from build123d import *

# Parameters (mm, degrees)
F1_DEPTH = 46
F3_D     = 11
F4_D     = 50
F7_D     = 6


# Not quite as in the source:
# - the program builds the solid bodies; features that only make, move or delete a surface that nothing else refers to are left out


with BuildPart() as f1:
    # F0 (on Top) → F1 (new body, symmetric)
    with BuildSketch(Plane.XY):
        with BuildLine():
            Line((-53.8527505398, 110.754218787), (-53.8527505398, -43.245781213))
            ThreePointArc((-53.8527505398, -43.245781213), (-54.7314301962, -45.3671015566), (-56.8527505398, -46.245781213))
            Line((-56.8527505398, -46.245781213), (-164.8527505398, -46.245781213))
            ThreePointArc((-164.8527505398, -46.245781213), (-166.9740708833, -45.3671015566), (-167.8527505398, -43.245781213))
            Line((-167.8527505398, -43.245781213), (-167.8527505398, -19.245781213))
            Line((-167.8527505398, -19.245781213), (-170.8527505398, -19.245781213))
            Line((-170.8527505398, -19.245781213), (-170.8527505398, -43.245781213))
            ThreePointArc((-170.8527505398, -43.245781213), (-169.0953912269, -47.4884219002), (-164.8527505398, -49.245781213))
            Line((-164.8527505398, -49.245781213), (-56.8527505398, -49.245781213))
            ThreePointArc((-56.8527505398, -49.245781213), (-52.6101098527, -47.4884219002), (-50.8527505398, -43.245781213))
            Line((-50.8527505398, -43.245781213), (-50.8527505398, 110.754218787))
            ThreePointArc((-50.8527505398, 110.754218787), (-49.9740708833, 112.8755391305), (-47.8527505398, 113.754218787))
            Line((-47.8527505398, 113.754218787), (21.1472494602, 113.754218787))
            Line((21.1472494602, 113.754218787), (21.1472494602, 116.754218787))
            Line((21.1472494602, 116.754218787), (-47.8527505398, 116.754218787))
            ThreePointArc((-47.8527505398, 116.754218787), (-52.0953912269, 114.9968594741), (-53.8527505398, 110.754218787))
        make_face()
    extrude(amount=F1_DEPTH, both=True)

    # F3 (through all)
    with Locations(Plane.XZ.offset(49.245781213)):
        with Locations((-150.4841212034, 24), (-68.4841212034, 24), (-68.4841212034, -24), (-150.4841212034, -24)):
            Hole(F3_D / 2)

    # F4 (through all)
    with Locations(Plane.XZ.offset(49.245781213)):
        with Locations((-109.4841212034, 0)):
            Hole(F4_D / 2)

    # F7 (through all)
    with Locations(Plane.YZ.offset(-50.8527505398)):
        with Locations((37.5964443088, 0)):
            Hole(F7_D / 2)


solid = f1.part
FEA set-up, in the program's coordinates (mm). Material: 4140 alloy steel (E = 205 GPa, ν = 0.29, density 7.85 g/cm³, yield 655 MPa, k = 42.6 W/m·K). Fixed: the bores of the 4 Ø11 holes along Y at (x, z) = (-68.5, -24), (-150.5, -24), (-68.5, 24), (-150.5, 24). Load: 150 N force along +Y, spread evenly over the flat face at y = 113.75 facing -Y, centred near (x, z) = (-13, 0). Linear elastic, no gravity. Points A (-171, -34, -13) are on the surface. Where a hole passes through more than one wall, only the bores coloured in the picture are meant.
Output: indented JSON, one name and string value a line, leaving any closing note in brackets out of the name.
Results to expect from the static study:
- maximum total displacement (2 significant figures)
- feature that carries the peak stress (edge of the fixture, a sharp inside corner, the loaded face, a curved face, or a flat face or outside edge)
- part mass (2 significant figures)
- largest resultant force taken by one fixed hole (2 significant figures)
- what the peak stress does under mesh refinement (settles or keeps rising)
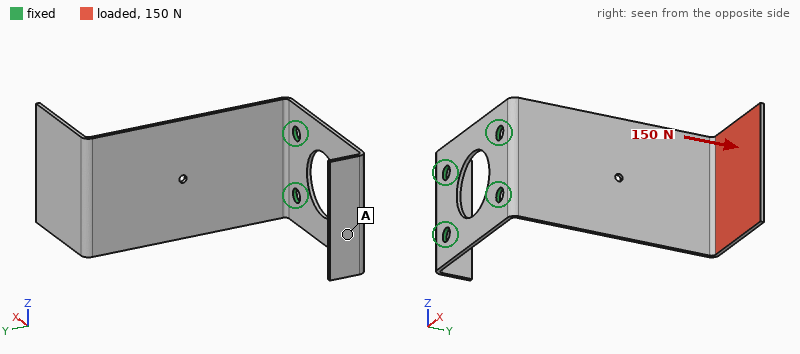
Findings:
{
  "maximum total displacement": "2.8 mm",
  "feature that carries the peak stress": "edge of the fixture",
  "part mass": "760 g",
  "largest resultant force taken by one fixed hole": "79 N",
  "what the peak stress does under mesh refinement": "keeps rising"
}
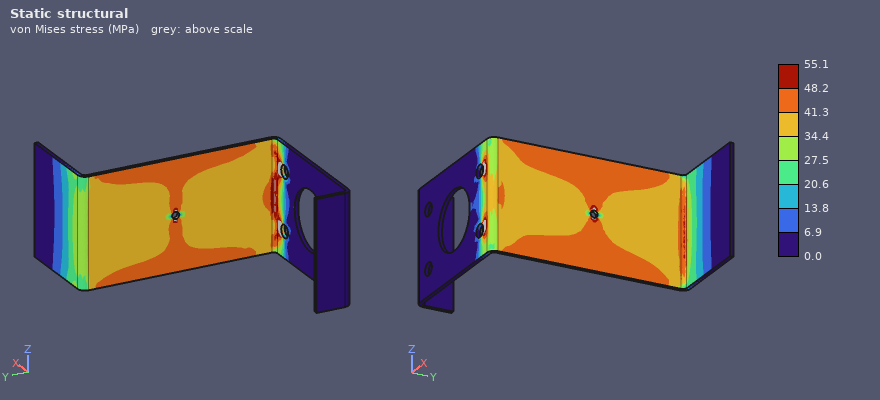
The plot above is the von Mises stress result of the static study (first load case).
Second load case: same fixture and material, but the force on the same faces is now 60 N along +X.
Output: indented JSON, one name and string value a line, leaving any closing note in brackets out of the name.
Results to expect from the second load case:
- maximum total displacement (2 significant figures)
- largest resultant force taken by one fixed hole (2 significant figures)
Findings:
{
  "maximum total displacement": "2.8 mm",
  "largest resultant force taken by one fixed hole": "44 N"
}
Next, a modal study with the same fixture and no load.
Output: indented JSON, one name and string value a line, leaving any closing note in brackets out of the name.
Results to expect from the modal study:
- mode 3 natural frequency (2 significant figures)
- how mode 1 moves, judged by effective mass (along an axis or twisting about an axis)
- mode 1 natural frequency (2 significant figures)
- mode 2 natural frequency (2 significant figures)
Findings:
{
  "mode 3 natural frequency": "230 Hz",
  "how mode 1 moves, judged by effective mass": "along X",
  "mode 1 natural frequency": "49 Hz",
  "mode 2 natural frequency": "160 Hz"
}
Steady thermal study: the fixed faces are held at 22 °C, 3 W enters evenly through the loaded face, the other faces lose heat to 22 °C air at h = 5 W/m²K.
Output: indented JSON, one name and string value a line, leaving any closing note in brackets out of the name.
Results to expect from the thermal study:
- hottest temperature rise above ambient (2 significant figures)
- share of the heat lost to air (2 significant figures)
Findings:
{
  "hottest temperature rise above ambient": "25 K",
  "share of the heat lost to air": "73 %"
}
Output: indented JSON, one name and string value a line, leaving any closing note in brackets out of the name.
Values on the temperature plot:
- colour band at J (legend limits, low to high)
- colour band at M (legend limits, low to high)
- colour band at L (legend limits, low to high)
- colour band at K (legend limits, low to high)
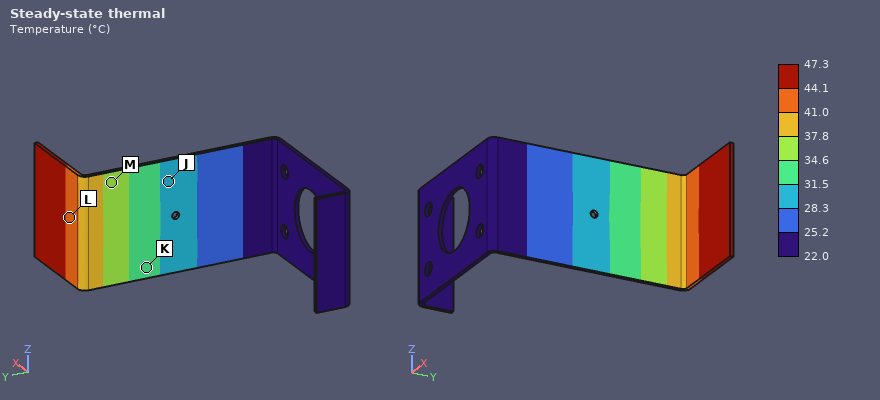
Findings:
{
  "colour band at J": "28.3 to 31.5 °C",
  "colour band at M": "34.6 to 37.8 °C",
  "colour band at L": "41.0 to 44.1 °C",
  "colour band at K": "31.5 to 34.6 °C"
}
